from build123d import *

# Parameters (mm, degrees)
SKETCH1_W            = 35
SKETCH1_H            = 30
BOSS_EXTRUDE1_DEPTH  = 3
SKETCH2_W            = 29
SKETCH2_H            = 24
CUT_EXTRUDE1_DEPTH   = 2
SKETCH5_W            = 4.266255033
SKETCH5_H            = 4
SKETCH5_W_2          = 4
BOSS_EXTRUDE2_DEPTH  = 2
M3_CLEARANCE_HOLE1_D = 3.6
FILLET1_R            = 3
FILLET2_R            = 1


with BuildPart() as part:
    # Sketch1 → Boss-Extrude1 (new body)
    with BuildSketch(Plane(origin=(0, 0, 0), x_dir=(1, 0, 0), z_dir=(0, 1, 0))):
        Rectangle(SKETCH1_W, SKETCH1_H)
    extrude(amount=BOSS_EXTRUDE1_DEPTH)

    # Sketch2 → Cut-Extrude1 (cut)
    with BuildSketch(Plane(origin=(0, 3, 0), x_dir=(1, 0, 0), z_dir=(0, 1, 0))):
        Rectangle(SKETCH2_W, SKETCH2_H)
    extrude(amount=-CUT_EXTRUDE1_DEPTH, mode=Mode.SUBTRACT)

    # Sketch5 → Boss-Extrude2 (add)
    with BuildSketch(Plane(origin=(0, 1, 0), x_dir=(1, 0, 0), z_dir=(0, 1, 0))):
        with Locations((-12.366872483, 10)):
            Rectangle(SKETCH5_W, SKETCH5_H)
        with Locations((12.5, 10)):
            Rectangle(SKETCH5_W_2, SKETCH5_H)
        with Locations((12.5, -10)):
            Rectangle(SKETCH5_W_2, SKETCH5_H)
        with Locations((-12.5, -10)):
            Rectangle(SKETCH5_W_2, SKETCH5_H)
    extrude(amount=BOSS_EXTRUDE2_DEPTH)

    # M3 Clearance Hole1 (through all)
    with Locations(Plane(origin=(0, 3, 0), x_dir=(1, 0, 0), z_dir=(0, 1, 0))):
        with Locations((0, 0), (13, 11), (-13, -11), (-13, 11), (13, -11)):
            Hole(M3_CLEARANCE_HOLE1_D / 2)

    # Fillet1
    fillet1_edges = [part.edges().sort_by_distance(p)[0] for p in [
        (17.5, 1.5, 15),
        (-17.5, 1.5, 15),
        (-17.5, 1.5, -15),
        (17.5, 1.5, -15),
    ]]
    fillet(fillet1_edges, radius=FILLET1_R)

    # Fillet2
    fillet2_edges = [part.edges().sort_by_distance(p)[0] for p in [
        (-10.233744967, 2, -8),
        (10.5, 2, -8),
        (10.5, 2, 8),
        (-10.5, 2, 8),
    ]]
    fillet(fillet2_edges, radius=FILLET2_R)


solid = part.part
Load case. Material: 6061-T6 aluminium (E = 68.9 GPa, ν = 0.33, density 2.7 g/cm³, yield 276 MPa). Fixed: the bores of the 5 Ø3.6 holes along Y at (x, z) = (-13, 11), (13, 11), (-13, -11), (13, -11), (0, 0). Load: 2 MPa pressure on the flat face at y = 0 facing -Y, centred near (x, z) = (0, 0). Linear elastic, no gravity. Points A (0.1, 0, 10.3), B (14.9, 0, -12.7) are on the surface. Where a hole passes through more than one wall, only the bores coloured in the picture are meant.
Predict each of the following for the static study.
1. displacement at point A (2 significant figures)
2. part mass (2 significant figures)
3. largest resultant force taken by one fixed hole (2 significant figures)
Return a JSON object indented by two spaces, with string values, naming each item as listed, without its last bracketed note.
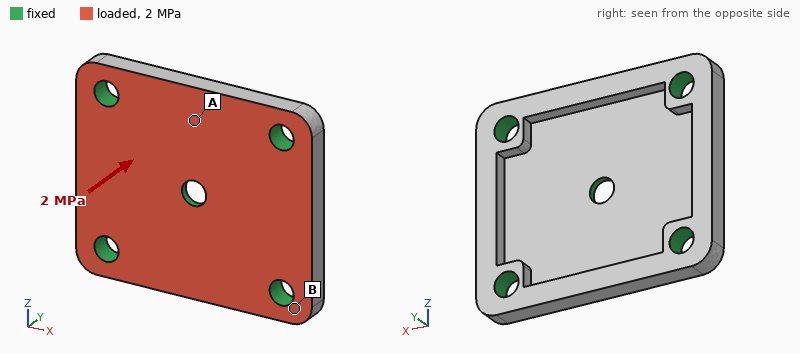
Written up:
{
  "displacement at point A": "32 µm",
  "part mass": "4.7 g",
  "largest resultant force taken by one fixed hole": "420 N"
}
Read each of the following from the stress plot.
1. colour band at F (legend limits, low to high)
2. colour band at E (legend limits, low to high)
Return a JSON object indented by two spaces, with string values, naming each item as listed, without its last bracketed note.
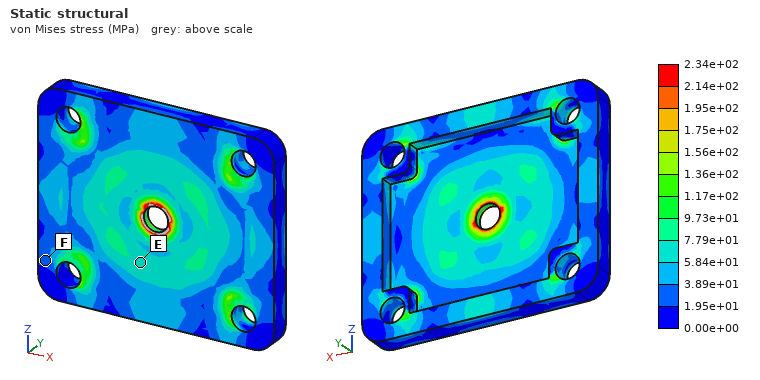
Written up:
{
  "colour band at F": "1.95e+01 to 3.89e+01 MPa",
  "colour band at E": "5.84e+01 to 7.79e+01 MPa"
}
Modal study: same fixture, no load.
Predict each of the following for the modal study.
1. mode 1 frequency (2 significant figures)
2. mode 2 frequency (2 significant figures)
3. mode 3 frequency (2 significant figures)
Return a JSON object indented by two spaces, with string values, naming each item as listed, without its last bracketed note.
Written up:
{
  "mode 1 frequency": "23 kHz",
  "mode 2 frequency": "23 kHz",
  "mode 3 frequency": "27 kHz"
}
